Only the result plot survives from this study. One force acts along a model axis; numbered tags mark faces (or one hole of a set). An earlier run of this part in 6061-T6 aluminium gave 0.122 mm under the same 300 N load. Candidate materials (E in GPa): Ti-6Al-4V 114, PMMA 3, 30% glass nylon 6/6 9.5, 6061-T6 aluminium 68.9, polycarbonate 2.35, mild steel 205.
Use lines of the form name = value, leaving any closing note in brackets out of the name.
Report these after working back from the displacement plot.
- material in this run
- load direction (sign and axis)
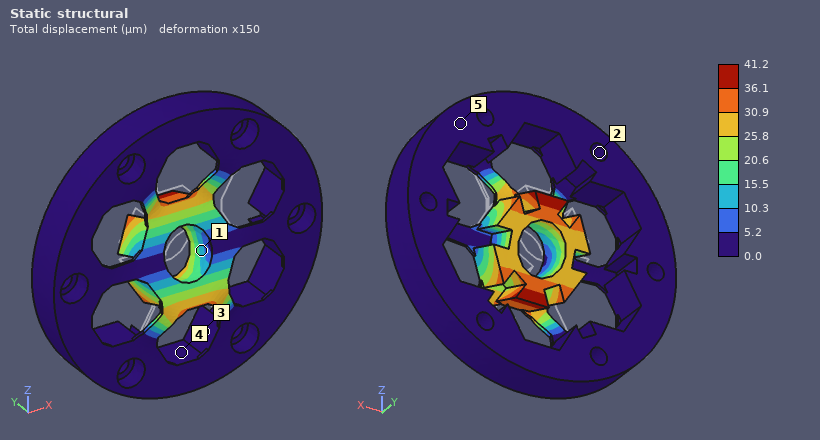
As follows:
material in this run = mild steel
load direction = -Z
